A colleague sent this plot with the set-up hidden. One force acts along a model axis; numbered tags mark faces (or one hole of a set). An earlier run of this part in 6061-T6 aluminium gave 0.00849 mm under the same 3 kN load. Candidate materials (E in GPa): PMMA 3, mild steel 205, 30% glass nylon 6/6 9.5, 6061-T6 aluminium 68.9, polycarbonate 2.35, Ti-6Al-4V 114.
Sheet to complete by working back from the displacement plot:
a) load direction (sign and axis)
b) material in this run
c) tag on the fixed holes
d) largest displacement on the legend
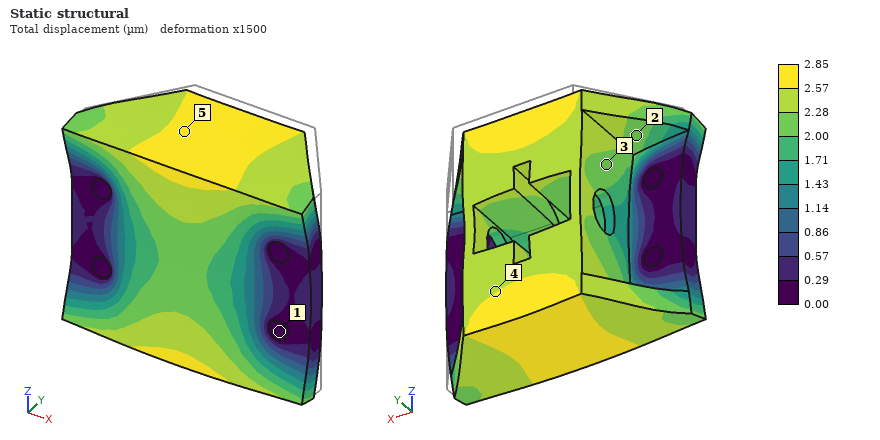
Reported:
-Y
mild steel
1
2.85 µm
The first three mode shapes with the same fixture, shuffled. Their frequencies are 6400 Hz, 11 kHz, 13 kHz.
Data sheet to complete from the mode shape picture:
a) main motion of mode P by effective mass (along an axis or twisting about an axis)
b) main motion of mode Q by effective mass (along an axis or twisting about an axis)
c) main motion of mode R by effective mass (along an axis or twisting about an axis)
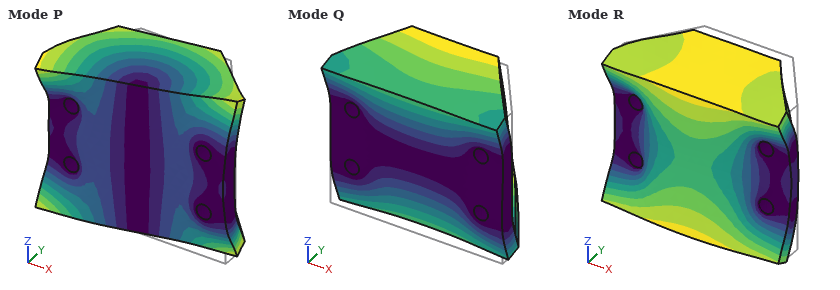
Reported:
along X
along Z
along Y
